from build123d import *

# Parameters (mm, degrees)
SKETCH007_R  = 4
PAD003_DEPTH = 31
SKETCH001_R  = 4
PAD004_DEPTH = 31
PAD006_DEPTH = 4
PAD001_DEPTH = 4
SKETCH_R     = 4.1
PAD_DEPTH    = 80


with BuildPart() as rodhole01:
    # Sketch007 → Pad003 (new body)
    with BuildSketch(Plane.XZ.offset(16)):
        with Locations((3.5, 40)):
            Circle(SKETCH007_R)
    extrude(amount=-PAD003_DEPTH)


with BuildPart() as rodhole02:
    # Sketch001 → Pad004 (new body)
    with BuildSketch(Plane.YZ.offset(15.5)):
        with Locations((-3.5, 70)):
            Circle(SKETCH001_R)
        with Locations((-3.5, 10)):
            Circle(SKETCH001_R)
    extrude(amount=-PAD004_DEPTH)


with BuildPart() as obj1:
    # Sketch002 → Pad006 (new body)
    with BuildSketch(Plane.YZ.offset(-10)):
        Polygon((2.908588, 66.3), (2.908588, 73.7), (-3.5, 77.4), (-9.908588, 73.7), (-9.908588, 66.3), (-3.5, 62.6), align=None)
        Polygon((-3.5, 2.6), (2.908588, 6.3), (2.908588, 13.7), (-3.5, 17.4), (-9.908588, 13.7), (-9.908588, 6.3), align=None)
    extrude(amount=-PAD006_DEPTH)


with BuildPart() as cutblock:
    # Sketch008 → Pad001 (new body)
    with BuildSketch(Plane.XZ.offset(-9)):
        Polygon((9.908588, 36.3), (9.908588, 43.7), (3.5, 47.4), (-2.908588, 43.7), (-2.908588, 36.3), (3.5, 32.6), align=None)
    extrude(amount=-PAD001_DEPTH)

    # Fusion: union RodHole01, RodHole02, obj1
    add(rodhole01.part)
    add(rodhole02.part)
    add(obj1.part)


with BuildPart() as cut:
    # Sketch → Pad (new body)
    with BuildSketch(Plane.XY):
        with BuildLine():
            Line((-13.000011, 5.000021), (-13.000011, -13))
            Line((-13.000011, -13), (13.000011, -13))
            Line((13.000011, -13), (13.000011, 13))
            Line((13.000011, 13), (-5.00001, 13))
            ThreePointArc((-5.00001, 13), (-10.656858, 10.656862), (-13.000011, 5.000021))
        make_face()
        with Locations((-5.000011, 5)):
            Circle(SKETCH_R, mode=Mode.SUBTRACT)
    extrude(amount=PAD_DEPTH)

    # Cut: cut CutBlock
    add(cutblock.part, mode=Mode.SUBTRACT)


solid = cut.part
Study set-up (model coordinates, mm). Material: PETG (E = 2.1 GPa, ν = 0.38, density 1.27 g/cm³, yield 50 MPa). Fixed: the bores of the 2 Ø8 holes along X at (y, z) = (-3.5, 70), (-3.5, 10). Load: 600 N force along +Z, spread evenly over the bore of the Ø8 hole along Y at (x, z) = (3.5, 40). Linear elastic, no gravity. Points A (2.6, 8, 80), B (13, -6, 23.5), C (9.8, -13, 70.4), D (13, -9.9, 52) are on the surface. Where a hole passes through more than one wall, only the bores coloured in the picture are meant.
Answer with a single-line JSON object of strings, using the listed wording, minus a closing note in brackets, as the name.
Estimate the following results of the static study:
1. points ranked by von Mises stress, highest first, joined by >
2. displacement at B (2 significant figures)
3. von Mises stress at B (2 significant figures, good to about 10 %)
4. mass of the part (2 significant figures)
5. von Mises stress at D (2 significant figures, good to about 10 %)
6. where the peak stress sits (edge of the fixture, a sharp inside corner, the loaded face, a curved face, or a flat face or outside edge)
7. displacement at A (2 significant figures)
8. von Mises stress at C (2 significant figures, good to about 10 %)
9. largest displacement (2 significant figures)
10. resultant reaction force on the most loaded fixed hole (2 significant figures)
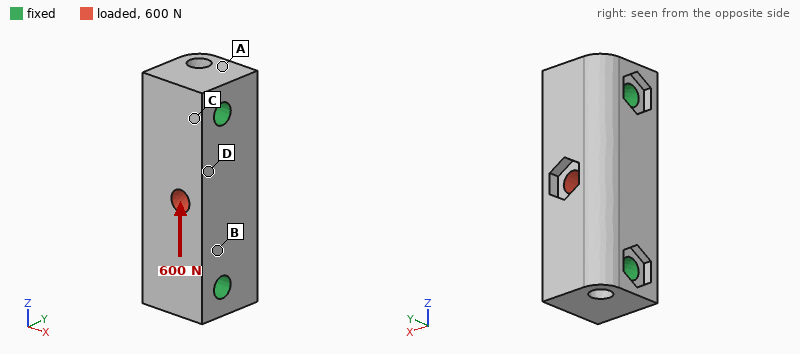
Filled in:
{"points ranked by von Mises stress, highest first, joined by >": "B > D > C > A", "displacement at B": "4.4 µm", "von Mises stress at B": "0.80 MPa", "mass of the part": "56 g", "von Mises stress at D": "0.59 MPa", "where the peak stress sits": "the loaded face", "displacement at A": "3.5 µm", "von Mises stress at C": "0.32 MPa", "largest displacement": "12 µm", "resultant reaction force on the most loaded fixed hole": "300 N"}
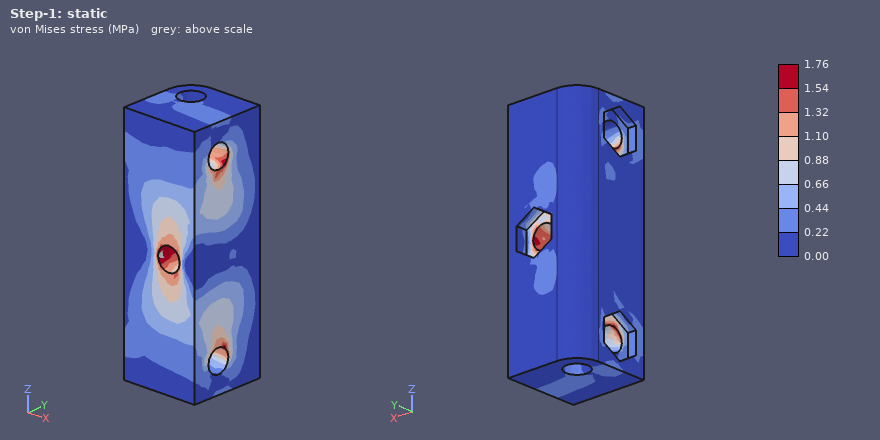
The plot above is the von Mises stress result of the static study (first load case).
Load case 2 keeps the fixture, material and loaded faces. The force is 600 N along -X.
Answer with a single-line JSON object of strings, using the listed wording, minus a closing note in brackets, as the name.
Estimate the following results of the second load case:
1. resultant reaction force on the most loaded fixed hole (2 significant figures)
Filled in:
{"resultant reaction force on the most loaded fixed hole": "300 N"}
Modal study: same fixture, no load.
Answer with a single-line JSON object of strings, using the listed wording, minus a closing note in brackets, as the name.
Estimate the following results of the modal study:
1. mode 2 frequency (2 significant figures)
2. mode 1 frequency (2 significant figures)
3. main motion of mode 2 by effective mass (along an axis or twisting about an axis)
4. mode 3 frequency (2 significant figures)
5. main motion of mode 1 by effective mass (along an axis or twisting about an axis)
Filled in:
{"mode 2 frequency": "4800 Hz", "mode 1 frequency": "4200 Hz", "main motion of mode 2 by effective mass": "along X", "mode 3 frequency": "5700 Hz", "main motion of mode 1 by effective mass": "along Y"}
